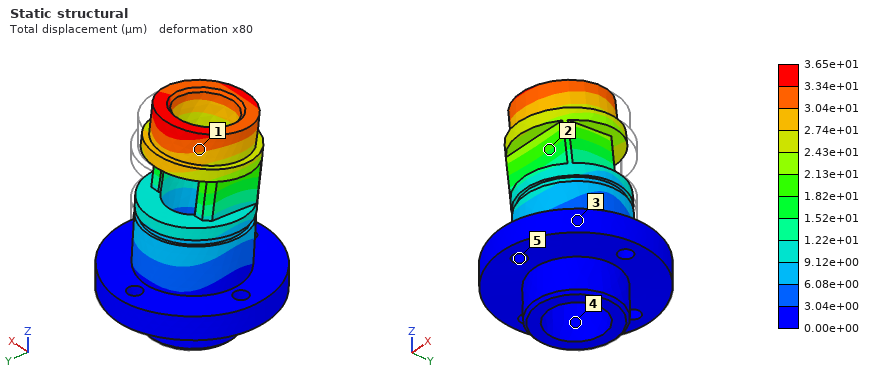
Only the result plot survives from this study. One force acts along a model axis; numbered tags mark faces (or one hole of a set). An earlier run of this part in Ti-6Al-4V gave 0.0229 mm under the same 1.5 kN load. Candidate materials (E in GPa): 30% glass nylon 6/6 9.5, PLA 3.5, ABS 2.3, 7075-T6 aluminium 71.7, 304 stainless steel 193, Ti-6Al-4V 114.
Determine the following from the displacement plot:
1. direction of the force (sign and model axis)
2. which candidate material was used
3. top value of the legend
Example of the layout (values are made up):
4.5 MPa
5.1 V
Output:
-Y
7075-T6 aluminium
3.65e+01 µm
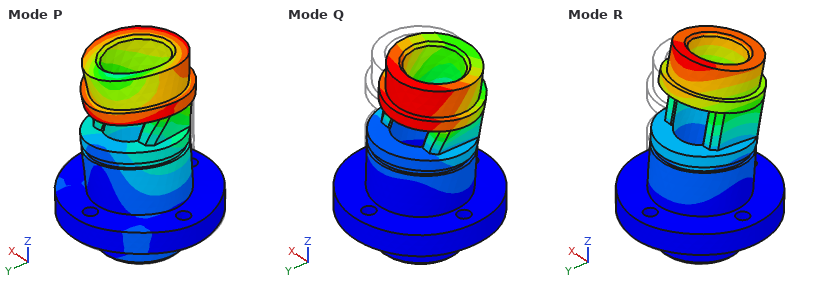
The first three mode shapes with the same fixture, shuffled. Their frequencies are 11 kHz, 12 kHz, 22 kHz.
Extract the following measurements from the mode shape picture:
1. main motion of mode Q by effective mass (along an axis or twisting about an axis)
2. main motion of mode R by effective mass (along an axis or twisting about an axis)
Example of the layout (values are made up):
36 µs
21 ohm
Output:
along X
along Y
